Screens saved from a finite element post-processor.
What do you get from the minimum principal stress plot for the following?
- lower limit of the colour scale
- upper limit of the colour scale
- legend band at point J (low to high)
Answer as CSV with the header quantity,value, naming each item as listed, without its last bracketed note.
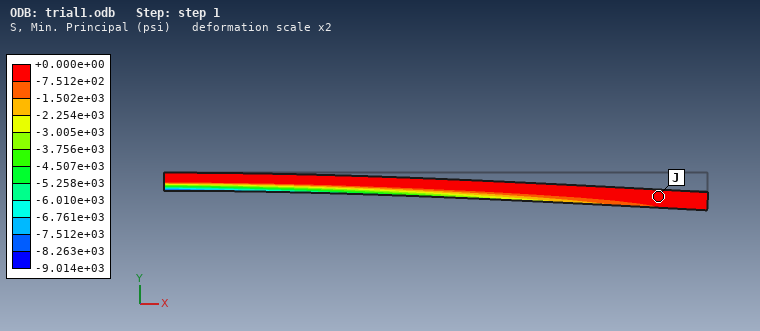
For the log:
quantity,value
lower limit of the colour scale,-9.014e+03 psi
upper limit of the colour scale,+0.000e+00 psi
legend band at point J,-7.512e+02 to +0.000e+00 psi
